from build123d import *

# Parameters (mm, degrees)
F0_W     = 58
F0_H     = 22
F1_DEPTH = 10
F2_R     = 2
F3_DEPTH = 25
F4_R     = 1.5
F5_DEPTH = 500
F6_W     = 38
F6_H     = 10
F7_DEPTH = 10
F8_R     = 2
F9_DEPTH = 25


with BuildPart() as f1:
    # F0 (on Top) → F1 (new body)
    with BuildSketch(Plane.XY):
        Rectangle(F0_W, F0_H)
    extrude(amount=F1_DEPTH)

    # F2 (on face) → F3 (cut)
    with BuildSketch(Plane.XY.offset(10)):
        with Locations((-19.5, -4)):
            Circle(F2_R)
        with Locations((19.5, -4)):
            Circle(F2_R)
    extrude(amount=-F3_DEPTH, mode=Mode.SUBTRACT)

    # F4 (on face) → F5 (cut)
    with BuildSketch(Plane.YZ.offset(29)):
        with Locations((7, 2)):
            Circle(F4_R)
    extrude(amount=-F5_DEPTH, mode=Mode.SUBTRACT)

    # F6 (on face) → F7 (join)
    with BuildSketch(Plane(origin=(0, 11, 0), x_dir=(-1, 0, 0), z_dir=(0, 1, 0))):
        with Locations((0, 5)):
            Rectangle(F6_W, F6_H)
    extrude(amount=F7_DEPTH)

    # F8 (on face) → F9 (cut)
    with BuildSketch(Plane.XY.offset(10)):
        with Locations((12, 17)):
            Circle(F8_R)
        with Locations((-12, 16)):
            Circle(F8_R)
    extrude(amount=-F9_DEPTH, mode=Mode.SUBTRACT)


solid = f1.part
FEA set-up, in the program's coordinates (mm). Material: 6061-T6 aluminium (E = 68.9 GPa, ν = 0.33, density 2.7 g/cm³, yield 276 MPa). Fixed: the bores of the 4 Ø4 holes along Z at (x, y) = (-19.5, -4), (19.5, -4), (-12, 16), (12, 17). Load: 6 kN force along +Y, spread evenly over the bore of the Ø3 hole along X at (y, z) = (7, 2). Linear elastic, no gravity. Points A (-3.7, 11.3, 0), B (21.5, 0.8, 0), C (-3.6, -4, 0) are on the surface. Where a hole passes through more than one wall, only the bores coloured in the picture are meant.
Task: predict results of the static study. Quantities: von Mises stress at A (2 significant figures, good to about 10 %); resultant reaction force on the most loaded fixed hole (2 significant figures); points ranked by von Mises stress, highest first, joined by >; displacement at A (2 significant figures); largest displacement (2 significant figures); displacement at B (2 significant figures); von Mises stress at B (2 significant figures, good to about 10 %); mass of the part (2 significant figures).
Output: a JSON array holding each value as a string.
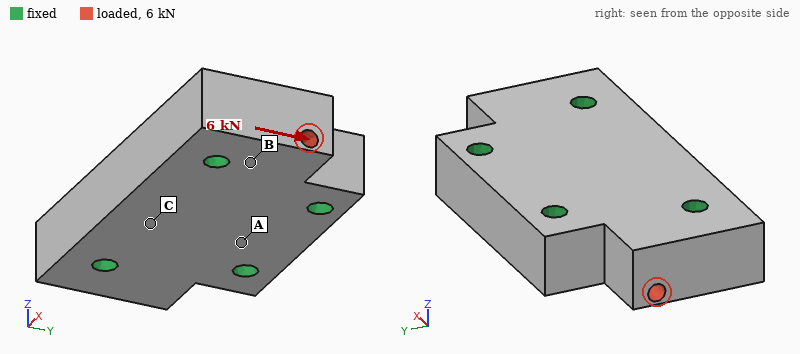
["12 MPa", "1.6 kN", "B > A > C", "2.4 µm", "6.5 µm", "1.4 µm", "24 MPa", "42 g"]
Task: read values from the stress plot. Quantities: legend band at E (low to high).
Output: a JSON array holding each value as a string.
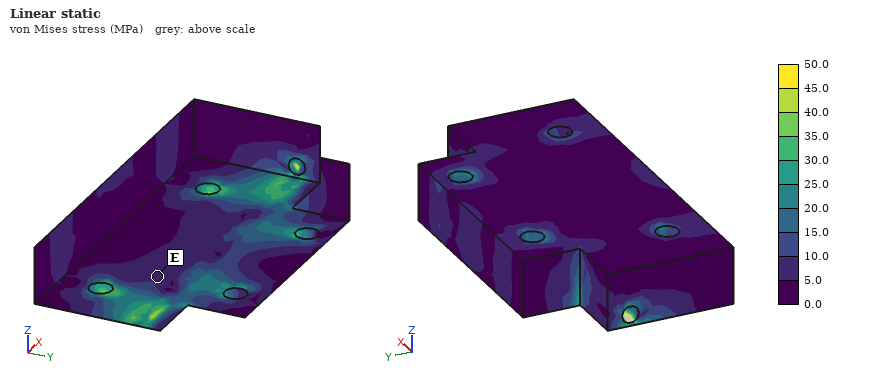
["5.0 to 10.0 MPa"]
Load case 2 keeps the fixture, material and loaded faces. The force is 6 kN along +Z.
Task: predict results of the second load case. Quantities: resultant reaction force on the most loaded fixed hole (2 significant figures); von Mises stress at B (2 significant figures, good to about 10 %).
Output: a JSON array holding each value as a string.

["1.6 kN", "23 MPa"]
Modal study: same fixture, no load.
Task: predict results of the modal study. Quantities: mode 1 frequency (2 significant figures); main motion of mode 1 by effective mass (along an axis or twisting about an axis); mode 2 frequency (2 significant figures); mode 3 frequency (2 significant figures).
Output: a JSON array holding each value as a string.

["27 kHz", "along Z", "37 kHz", "38 kHz"]
